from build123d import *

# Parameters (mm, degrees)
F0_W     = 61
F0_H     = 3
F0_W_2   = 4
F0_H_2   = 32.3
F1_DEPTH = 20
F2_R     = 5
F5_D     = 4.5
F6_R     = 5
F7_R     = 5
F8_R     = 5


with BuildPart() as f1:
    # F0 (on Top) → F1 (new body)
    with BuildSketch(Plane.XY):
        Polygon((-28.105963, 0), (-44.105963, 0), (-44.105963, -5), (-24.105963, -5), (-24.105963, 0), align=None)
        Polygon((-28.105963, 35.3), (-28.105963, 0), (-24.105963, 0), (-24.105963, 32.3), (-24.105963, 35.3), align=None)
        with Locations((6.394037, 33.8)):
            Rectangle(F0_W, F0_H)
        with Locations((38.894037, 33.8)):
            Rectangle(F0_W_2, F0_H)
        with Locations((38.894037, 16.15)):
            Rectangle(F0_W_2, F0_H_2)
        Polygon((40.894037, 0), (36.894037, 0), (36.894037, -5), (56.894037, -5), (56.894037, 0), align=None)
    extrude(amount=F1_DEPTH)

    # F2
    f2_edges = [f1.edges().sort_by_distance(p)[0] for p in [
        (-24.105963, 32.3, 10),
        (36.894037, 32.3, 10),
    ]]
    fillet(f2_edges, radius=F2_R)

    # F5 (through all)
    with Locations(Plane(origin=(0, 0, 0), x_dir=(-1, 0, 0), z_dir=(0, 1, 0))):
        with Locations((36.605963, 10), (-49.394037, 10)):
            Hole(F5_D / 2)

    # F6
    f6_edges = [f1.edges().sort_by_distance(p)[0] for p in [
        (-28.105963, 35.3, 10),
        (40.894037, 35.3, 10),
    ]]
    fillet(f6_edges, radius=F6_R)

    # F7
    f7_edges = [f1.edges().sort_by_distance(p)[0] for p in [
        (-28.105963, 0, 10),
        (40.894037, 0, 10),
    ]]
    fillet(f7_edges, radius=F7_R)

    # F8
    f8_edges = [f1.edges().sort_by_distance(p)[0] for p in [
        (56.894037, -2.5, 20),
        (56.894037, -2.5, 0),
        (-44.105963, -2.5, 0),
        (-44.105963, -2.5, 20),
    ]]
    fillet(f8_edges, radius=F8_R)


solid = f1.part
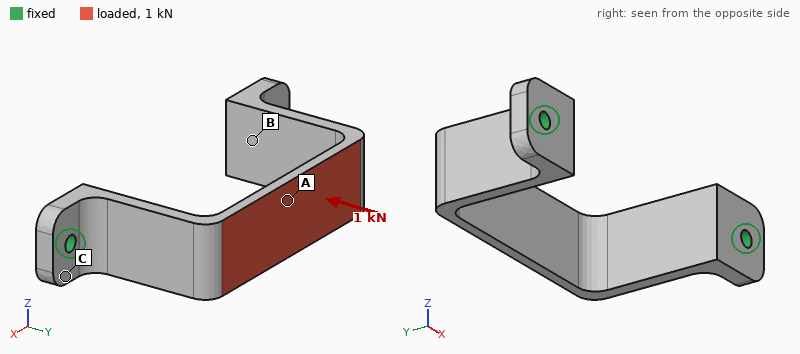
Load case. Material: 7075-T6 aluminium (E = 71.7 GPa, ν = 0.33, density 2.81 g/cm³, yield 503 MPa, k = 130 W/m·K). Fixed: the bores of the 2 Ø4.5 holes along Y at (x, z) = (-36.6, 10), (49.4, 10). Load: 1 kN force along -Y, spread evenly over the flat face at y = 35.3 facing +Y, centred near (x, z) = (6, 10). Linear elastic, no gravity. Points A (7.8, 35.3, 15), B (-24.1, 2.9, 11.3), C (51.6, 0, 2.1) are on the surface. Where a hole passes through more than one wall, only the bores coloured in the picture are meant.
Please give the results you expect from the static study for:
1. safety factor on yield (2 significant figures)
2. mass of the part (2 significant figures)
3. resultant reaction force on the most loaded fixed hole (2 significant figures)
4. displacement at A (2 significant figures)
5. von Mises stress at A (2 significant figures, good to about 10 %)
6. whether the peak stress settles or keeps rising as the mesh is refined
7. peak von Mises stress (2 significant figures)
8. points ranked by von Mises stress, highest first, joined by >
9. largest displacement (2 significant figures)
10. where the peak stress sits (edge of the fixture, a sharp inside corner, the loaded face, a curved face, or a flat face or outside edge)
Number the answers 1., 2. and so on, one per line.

1. 4.9
2. 37 g
3. 570 N
4. 0.24 mm
5. 95 MPa
6. settles
7. 100 MPa
8. A > B > C
9. 0.25 mm
10. a curved face
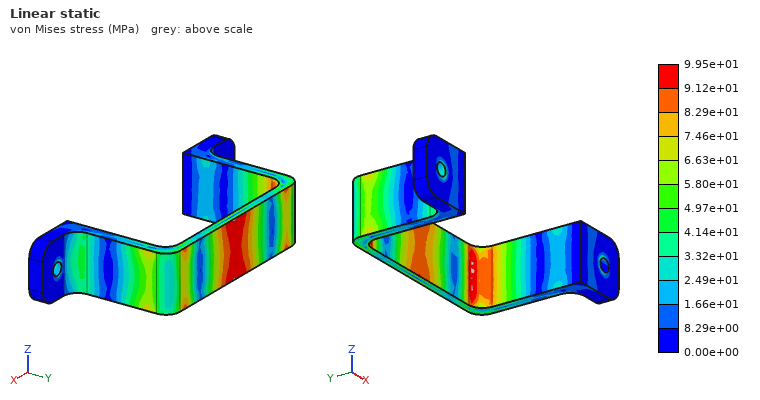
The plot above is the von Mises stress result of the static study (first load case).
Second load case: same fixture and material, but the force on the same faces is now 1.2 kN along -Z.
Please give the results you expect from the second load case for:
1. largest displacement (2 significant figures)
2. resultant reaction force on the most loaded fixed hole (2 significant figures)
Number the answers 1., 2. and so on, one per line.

1. 0.40 mm
2. 600 N
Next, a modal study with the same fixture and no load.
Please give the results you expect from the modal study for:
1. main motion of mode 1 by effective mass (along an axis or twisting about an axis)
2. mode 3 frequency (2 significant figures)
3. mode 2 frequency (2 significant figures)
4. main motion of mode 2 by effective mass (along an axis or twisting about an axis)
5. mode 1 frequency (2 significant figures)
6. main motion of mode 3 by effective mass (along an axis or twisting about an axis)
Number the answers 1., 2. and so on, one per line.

1. along X
2. 3300 Hz
3. 2300 Hz
4. along Z
5. 1800 Hz
6. twisting about Y
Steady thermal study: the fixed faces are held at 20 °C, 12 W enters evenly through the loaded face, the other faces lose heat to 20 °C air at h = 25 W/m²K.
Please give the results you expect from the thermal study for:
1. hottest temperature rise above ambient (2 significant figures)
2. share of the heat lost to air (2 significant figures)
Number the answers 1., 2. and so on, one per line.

1. 30 K
2. 18 %
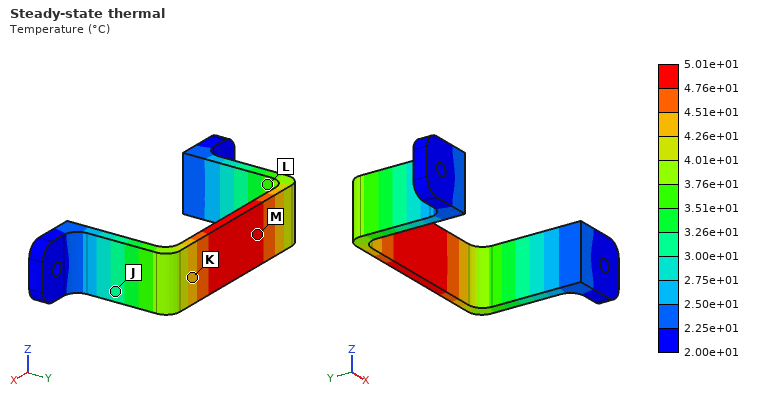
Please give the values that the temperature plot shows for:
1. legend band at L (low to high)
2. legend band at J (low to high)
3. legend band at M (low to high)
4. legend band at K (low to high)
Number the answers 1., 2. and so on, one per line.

1. 3.51e+01 to 3.76e+01 °C
2. 3.00e+01 to 3.26e+01 °C
3. 4.76e+01 to 5.01e+01 °C
4. 4.26e+01 to 4.51e+01 °C
